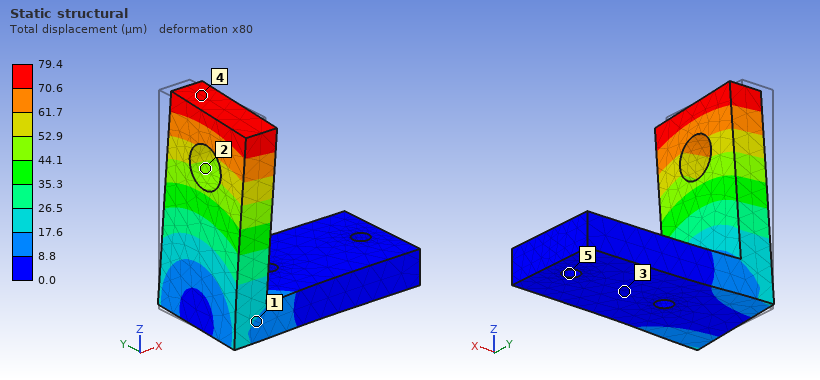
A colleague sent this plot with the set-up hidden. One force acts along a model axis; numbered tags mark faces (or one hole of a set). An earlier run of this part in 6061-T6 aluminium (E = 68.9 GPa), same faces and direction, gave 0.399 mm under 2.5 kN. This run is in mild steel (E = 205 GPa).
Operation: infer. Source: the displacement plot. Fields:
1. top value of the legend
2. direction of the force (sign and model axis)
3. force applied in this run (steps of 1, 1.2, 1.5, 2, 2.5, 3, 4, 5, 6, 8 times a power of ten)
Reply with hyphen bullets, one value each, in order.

- 79.4 µm
- -Y
- 1.5 kN
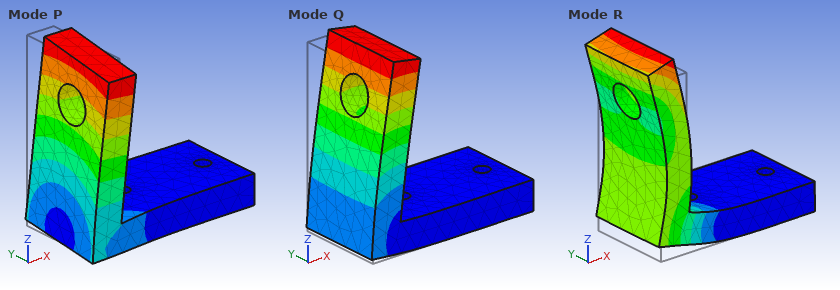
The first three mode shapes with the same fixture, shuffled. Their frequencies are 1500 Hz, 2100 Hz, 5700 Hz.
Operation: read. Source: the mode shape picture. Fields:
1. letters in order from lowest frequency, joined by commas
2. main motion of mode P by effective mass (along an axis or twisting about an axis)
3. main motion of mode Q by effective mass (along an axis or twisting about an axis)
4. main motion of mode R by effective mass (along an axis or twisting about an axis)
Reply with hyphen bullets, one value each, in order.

- Q, P, R
- along Y
- along X
- along Z
